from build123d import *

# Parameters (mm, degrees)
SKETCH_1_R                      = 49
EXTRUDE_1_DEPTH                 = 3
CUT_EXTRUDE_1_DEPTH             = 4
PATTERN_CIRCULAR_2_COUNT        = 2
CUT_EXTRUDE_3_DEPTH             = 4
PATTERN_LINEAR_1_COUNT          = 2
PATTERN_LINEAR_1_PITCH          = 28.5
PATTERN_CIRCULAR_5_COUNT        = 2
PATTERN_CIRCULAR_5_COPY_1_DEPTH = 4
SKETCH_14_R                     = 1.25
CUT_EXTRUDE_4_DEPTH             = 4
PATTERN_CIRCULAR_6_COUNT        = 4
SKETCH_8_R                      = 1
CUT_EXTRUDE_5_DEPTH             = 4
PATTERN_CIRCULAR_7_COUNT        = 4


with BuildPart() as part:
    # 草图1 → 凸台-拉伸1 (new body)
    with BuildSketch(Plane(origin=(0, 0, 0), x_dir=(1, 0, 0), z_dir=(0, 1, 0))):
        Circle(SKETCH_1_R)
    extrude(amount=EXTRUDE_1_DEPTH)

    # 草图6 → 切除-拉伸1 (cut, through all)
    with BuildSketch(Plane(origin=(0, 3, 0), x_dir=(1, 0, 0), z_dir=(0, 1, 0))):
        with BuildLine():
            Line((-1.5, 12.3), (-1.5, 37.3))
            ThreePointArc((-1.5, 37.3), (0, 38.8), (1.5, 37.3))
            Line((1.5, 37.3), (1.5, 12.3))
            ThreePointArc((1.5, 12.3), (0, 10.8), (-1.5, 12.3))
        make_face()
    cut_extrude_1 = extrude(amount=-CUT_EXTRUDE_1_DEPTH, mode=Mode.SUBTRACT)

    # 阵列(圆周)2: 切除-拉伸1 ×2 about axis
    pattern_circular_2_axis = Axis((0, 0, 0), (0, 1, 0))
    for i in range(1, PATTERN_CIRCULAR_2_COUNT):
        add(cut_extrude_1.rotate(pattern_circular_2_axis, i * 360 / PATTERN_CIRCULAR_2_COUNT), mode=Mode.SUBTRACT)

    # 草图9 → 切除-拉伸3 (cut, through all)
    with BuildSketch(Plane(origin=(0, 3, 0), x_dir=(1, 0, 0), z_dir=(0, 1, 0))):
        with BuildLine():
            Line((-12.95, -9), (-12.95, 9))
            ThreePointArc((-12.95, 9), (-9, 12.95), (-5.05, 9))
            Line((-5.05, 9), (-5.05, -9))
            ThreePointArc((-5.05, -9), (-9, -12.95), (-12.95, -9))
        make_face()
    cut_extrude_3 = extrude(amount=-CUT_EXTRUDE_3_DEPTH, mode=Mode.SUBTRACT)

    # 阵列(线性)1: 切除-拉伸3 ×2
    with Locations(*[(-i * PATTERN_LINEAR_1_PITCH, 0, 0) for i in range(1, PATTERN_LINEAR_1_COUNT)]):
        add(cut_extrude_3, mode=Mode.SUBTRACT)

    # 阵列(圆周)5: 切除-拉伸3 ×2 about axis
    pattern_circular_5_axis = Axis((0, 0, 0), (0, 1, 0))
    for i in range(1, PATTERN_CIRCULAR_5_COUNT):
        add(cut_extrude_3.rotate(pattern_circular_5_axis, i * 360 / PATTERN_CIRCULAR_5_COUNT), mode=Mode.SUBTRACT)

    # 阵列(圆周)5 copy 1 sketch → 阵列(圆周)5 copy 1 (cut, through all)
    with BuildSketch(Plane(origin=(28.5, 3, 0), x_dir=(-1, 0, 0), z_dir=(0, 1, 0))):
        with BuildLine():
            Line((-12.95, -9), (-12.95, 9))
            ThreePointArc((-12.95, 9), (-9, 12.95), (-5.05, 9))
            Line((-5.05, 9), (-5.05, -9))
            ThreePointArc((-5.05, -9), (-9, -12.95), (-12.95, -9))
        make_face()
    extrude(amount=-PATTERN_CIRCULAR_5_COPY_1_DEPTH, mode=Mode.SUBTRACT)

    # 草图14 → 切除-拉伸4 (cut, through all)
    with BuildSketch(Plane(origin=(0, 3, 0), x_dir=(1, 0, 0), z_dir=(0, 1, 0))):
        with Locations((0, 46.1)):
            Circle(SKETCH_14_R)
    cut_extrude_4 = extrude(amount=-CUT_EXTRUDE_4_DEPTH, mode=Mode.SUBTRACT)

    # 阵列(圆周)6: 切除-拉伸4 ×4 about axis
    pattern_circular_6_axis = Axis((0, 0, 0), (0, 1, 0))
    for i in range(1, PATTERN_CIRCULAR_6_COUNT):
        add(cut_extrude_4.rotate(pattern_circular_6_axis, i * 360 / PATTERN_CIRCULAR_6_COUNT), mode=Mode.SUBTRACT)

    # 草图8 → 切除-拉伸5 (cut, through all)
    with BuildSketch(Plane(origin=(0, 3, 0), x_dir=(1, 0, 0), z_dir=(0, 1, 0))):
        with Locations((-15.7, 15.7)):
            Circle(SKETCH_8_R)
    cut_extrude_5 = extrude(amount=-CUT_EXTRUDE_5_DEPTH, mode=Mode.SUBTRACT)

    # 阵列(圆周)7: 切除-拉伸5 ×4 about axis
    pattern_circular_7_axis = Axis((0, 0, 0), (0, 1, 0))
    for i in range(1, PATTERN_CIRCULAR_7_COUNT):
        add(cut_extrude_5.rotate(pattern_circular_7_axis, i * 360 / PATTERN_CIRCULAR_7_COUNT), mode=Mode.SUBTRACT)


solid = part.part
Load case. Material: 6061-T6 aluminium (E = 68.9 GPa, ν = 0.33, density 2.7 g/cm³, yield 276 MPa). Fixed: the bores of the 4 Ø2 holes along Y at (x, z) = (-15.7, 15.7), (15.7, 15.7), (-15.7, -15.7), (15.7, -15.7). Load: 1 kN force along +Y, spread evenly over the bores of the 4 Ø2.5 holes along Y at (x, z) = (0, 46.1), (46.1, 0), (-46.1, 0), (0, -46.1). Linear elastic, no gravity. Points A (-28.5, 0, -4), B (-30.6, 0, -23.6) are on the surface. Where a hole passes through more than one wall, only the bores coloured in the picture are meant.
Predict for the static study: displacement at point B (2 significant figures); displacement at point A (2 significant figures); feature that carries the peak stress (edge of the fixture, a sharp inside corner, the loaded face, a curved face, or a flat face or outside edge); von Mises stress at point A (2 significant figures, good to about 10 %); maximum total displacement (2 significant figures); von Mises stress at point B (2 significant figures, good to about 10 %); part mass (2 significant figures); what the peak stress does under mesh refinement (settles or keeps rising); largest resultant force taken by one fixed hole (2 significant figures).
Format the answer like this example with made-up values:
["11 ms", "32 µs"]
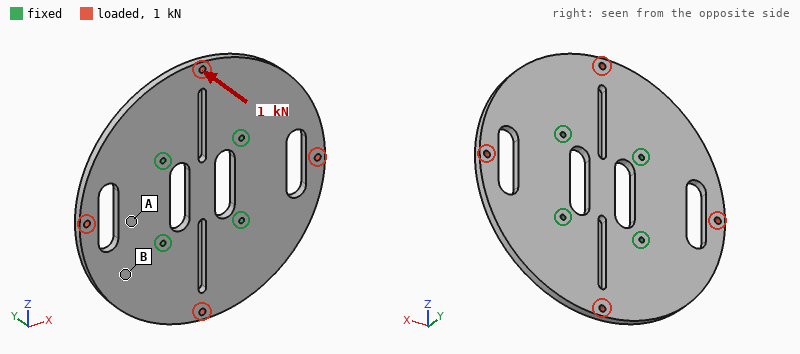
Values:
["0.11 mm", "0.063 mm", "edge of the fixture", "23 MPa", "0.41 mm", "59 MPa", "53 g", "keeps rising", "250 N"]
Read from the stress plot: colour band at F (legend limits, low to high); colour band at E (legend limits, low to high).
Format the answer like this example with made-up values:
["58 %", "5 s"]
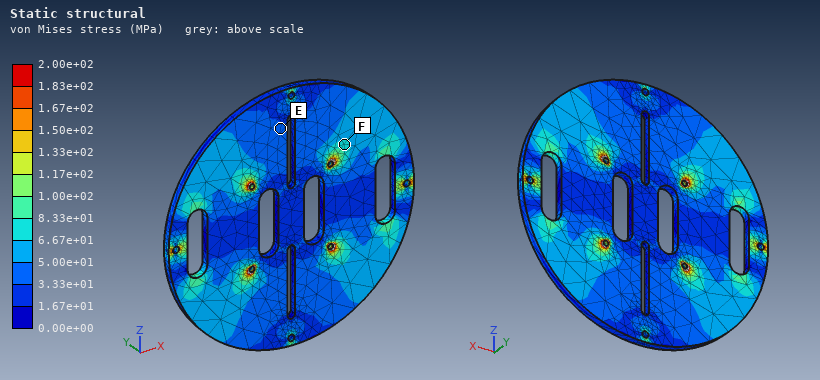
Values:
["6.67e+01 to 8.33e+01 MPa", "3.33e+01 to 5.00e+01 MPa"]
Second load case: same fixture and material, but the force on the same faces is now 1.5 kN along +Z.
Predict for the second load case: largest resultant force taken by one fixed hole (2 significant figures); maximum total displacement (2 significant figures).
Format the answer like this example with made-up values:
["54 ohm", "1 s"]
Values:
["390 N", "8.3 µm"]
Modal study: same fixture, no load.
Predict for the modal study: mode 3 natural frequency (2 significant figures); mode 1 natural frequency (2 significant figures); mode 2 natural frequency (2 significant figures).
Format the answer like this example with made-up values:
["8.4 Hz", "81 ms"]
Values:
["2400 Hz", "2200 Hz", "2400 Hz"]
